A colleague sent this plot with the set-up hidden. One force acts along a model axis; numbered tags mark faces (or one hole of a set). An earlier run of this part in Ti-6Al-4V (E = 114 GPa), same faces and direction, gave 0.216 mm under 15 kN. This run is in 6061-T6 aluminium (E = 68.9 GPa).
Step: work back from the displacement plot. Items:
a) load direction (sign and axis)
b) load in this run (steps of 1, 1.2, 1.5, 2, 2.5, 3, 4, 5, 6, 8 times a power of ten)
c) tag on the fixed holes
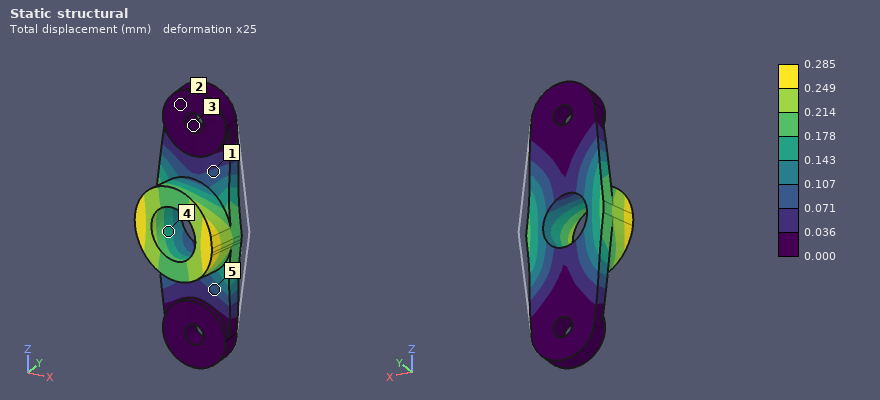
-X
12 kN
3
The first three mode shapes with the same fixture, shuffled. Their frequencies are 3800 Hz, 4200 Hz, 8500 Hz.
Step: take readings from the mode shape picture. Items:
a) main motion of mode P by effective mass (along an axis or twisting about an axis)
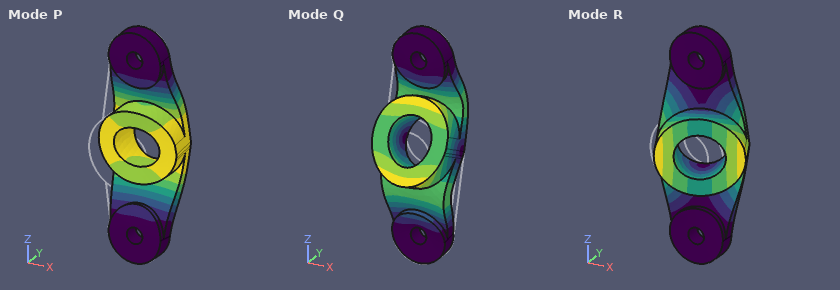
along Y
